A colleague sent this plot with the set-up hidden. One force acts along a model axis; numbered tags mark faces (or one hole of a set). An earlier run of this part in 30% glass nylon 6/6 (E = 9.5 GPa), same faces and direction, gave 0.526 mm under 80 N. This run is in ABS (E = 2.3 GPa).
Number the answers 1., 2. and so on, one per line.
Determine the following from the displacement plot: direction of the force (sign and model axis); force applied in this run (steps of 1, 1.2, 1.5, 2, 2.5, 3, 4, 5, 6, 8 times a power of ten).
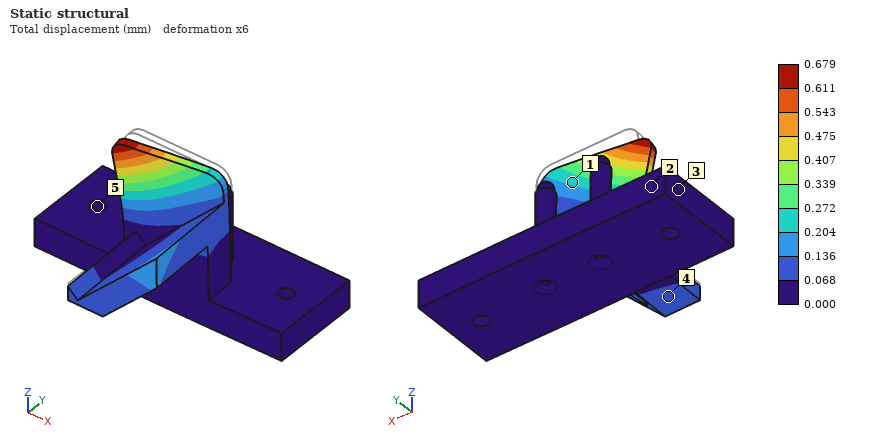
1. -Y
2. 25 N
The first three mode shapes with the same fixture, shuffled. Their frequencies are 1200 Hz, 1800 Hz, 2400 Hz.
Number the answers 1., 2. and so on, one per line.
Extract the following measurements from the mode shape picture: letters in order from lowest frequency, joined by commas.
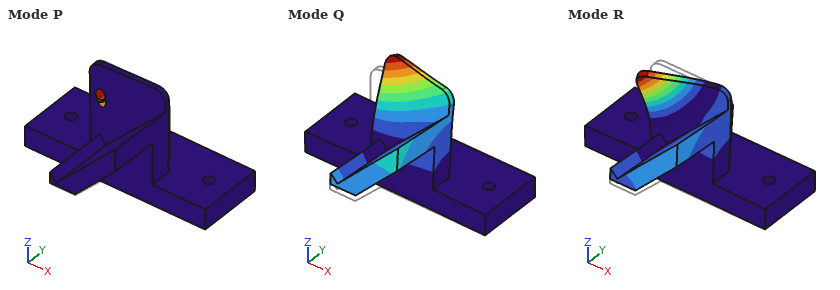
1. Q, R, P
